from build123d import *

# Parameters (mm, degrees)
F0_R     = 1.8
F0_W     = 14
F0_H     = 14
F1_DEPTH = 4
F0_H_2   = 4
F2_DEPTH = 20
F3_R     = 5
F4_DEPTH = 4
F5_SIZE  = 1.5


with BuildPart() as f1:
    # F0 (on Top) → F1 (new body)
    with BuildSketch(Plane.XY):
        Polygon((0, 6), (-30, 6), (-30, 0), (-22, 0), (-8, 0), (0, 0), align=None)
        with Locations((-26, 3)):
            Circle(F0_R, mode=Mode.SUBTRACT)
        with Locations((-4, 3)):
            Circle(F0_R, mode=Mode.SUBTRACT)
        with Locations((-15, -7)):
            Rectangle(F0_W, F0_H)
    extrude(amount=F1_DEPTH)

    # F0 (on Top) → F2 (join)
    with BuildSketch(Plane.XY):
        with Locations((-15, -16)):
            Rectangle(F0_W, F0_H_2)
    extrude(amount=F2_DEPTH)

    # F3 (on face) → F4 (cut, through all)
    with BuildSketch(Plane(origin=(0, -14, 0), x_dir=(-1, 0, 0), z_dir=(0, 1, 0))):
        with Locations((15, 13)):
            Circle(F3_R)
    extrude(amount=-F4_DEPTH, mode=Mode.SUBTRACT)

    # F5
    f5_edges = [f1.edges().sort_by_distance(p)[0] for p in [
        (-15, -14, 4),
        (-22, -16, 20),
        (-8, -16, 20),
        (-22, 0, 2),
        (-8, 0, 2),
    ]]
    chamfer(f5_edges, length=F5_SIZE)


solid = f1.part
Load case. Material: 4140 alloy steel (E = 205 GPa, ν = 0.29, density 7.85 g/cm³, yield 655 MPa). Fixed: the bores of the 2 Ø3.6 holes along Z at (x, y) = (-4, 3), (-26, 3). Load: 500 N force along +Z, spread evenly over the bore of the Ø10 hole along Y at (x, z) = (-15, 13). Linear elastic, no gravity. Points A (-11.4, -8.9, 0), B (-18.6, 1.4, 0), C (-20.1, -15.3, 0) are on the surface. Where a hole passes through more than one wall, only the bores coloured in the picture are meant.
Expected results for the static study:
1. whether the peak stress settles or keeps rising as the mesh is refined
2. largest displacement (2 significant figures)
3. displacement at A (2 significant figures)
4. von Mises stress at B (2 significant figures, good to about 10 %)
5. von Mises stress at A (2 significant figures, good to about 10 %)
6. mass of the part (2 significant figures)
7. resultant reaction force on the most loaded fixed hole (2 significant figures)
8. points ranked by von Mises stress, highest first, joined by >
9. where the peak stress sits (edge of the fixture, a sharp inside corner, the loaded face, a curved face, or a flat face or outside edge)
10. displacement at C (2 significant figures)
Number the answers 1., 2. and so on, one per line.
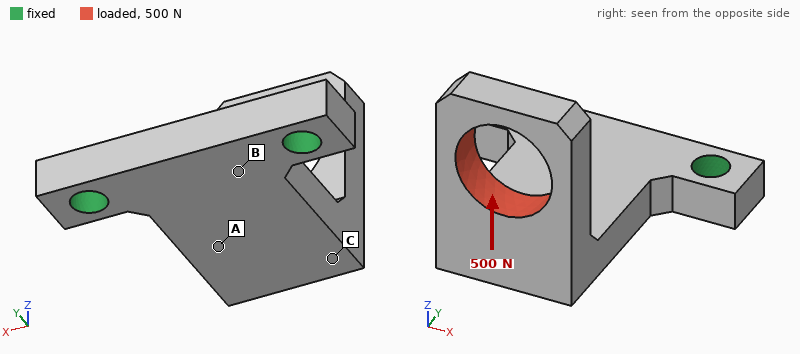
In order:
1. keeps rising
2. 0.19 mm
3. 0.062 mm
4. 150 MPa
5. 97 MPa
6. 18 g
7. 250 N
8. B > A > C
9. edge of the fixture
10. 0.11 mm
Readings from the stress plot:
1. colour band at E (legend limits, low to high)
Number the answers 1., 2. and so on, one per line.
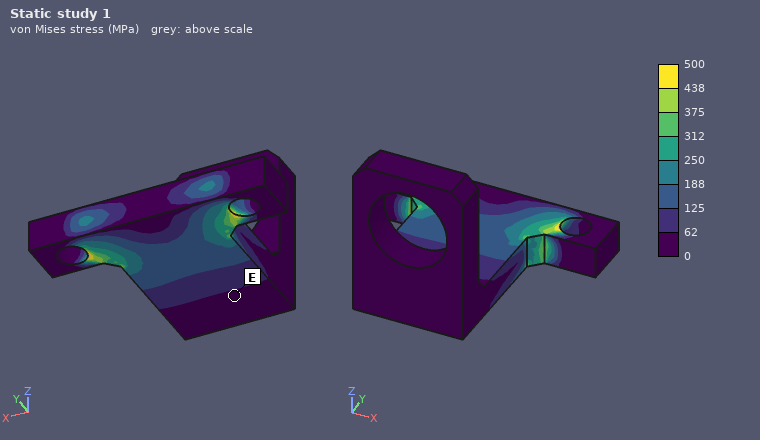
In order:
1. 0 to 62 MPa
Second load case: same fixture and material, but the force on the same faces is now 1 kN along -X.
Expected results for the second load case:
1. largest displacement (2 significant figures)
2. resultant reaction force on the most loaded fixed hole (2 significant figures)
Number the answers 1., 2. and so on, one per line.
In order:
1. 0.18 mm
2. 1.3 kN
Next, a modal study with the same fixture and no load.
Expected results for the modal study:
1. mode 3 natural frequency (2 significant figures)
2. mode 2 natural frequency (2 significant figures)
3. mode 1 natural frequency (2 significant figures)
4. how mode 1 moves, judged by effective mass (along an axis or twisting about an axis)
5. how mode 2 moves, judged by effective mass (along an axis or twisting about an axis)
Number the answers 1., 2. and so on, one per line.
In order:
1. 9500 Hz
2. 6700 Hz
3. 3200 Hz
4. along Z
5. along X
